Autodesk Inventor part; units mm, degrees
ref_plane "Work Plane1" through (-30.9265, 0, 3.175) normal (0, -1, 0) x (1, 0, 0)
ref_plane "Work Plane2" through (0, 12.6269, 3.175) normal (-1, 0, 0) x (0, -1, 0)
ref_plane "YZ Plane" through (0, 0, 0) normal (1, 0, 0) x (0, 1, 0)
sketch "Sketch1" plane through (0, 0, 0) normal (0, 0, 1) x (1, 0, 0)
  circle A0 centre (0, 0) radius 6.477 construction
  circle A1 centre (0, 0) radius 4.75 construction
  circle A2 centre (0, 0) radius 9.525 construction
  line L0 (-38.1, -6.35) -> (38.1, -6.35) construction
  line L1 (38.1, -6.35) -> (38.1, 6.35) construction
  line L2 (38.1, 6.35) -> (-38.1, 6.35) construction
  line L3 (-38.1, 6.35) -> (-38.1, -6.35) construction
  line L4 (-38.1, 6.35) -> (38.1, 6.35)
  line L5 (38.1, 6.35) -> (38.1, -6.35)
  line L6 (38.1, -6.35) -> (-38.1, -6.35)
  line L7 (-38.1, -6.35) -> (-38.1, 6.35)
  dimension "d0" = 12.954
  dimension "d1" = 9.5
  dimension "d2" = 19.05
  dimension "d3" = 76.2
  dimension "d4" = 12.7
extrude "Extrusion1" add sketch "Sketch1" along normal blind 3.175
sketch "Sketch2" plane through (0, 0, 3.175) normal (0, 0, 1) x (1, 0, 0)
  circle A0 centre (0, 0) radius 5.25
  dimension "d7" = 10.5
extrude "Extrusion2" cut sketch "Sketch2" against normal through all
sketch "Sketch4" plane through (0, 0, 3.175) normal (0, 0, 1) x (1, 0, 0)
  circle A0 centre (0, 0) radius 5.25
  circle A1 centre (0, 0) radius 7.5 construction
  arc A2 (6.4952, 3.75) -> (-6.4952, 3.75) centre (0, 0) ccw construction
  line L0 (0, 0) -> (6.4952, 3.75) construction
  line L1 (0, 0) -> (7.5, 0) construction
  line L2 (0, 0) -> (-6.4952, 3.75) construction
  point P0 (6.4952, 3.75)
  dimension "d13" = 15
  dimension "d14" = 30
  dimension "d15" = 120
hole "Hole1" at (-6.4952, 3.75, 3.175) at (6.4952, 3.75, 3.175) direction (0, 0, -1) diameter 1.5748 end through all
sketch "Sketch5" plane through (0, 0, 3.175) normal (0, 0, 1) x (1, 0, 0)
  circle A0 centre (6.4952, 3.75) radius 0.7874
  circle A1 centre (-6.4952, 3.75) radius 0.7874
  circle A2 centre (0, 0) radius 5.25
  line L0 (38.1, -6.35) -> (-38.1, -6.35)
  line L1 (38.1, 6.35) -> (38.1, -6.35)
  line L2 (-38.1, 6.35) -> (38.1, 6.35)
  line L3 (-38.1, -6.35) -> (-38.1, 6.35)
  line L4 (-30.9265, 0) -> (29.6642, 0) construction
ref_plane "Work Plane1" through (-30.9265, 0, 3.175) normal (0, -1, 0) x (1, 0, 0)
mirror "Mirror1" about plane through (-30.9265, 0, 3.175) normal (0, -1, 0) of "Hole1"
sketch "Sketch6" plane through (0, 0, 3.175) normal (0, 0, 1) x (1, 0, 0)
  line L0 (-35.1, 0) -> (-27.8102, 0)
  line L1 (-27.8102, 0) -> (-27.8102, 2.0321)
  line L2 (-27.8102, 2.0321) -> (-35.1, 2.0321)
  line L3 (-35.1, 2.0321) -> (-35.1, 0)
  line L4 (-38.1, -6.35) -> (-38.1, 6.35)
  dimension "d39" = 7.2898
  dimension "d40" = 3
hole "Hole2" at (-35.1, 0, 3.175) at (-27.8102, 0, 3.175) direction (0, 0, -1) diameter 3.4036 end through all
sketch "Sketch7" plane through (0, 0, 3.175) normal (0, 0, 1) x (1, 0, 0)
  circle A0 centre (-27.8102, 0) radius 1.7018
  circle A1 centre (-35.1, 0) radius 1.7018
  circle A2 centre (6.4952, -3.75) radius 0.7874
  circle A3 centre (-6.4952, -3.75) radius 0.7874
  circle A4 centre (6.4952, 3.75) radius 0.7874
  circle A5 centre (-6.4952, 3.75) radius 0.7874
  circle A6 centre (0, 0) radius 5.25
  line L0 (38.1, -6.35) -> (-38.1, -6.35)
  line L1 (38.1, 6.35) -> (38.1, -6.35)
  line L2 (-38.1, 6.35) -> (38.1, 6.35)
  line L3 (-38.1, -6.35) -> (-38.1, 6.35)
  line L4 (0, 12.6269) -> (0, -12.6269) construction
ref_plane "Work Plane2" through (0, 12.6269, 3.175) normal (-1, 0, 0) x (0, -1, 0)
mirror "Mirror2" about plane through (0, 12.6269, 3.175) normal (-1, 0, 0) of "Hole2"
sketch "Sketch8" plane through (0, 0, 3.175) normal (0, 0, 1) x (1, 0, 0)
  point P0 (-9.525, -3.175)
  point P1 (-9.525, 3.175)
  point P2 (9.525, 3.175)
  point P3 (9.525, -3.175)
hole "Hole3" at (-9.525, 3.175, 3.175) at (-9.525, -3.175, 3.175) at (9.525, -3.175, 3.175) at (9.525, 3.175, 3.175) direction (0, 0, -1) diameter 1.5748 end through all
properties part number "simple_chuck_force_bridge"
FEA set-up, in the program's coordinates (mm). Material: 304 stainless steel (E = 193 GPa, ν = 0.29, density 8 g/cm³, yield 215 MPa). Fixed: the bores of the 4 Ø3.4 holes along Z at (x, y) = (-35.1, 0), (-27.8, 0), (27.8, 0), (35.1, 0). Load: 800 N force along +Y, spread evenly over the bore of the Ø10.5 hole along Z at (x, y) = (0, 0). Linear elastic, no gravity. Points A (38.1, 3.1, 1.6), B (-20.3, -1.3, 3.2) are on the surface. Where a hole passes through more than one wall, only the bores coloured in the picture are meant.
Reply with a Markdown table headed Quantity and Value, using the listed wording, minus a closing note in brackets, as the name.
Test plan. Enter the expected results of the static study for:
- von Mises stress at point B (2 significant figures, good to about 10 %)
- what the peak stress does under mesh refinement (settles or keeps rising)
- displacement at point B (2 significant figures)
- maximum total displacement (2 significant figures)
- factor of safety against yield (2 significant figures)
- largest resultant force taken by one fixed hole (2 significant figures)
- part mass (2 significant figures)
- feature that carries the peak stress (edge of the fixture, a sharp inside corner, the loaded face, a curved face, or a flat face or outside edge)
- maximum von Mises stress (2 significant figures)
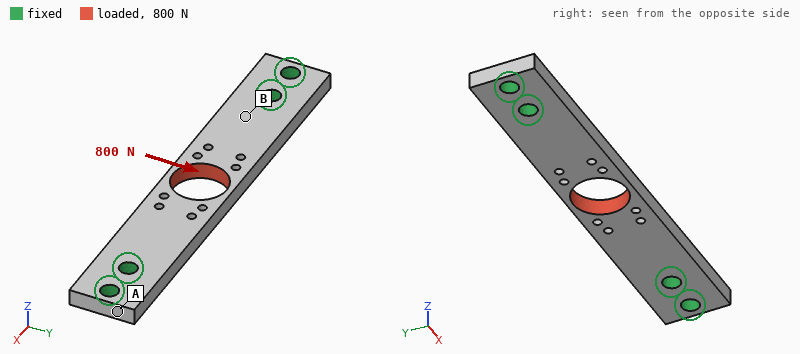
| Quantity | Value |
|---|---|
| von Mises stress at point B | 25 MPa |
| what the peak stress does under mesh refinement | settles |
| displacement at point B | 3.7 µm |
| maximum total displacement | 16 µm |
| factor of safety against yield | 1.8 |
| largest resultant force taken by one fixed hole | 760 N |
| part mass | 21 g |
| feature that carries the peak stress | the loaded face |
| maximum von Mises stress | 120 MPa |
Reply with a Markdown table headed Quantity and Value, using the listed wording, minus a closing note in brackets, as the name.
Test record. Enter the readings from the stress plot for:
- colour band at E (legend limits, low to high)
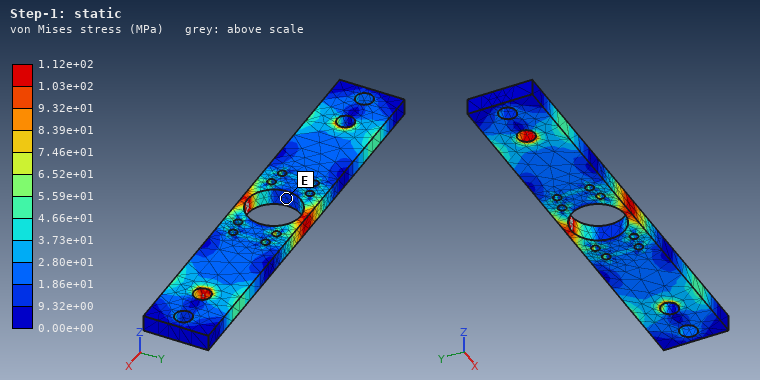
| Quantity | Value |
|---|---|
| colour band at E | 9.32e+00 to 1.86e+01 MPa |
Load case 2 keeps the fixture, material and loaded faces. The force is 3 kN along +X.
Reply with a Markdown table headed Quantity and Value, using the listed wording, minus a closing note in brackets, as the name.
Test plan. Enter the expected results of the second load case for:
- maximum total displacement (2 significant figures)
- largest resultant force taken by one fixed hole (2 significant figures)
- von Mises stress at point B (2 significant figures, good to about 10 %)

| Quantity | Value |
|---|---|
| maximum total displacement | 6.4 µm |
| largest resultant force taken by one fixed hole | 1.3 kN |
| von Mises stress at point B | 42 MPa |
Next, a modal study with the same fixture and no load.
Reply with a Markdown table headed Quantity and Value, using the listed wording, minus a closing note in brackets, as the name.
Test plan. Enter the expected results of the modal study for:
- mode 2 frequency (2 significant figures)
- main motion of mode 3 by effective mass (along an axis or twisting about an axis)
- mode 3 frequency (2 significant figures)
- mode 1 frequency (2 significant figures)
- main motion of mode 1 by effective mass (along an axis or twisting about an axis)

| Quantity | Value |
|---|---|
| mode 2 frequency | 13 kHz |
| main motion of mode 3 by effective mass | twisting about X |
| mode 3 frequency | 14 kHz |
| mode 1 frequency | 5400 Hz |
| main motion of mode 1 by effective mass | along Z |
